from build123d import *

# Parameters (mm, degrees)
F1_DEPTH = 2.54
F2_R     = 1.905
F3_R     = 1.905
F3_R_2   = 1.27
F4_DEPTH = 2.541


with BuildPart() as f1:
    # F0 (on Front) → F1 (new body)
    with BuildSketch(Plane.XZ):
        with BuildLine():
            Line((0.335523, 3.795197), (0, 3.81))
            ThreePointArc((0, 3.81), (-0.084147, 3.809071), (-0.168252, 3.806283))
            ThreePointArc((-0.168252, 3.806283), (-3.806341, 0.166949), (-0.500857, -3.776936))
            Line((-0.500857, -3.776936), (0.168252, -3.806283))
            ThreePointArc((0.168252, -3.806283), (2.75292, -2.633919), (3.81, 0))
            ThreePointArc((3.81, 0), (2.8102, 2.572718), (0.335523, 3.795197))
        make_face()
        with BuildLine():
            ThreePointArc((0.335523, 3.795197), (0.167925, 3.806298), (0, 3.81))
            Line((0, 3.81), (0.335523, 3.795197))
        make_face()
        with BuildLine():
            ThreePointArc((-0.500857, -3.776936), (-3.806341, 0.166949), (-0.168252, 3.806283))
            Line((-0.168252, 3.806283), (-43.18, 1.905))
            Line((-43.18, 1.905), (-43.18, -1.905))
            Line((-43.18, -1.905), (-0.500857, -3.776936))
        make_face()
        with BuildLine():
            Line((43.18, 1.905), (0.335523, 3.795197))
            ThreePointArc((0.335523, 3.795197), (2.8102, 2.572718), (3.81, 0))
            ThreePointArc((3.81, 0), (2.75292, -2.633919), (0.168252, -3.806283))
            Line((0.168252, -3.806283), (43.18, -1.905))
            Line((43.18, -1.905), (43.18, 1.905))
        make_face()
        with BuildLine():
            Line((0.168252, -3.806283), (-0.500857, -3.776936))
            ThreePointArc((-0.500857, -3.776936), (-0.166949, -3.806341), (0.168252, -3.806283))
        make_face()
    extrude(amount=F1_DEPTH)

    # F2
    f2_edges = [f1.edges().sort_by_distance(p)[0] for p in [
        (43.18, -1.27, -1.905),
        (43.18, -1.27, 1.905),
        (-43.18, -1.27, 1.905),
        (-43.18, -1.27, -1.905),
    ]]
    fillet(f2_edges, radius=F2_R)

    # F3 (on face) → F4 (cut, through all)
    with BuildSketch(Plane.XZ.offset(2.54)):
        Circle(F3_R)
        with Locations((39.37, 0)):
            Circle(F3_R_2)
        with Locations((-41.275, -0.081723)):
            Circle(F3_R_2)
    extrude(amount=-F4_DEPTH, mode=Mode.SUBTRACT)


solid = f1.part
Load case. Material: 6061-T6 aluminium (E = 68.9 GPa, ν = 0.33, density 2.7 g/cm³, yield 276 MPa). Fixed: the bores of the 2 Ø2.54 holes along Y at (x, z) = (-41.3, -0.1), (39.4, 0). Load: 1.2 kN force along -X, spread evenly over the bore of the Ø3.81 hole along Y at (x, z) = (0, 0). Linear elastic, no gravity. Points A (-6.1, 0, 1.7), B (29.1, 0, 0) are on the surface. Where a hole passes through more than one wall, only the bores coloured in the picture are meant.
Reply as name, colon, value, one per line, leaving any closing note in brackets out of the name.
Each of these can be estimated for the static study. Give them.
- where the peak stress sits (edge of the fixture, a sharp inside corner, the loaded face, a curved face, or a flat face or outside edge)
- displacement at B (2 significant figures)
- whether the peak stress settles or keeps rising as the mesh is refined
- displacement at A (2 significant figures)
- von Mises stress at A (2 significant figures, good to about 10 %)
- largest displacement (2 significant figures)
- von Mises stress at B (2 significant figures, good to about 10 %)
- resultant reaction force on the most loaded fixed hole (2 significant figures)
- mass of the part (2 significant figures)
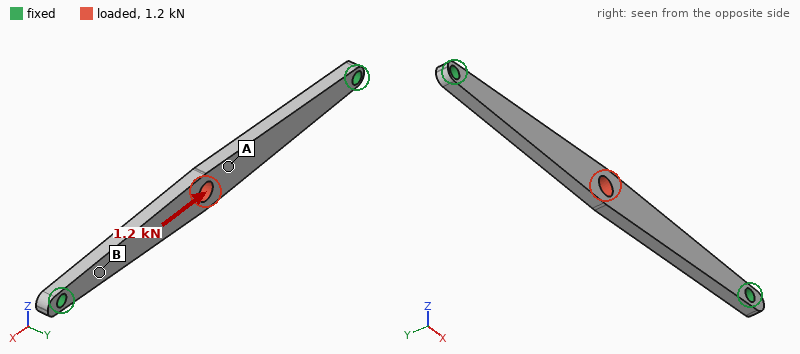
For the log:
where the peak stress sits: edge of the fixture
displacement at B: 7.3 µm
whether the peak stress settles or keeps rising as the mesh is refined: keeps rising
displacement at A: 21 µm
von Mises stress at A: 33 MPa
largest displacement: 24 µm
von Mises stress at B: 48 MPa
resultant reaction force on the most loaded fixed hole: 620 N
mass of the part: 3.2 g
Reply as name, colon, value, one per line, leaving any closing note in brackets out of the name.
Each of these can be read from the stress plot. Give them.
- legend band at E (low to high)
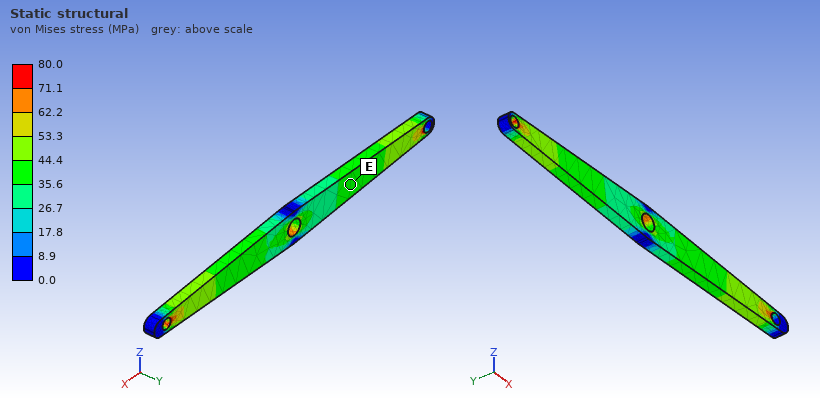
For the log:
legend band at E: 35.6 to 44.4 MPa
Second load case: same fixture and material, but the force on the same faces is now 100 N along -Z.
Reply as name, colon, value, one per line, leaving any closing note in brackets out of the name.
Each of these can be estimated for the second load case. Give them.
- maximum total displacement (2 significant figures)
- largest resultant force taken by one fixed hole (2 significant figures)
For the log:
maximum total displacement: 0.10 mm
largest resultant force taken by one fixed hole: 52 N
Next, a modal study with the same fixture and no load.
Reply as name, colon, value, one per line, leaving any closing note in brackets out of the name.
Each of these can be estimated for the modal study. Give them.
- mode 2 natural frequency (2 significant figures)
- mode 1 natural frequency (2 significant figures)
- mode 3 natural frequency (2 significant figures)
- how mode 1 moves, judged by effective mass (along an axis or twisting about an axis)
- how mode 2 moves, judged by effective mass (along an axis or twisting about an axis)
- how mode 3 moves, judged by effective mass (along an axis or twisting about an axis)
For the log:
mode 2 natural frequency: 3900 Hz
mode 1 natural frequency: 1900 Hz
mode 3 natural frequency: 5500 Hz
how mode 1 moves, judged by effective mass: along Y
how mode 2 moves, judged by effective mass: along Z
how mode 3 moves, judged by effective mass: twisting about Z
